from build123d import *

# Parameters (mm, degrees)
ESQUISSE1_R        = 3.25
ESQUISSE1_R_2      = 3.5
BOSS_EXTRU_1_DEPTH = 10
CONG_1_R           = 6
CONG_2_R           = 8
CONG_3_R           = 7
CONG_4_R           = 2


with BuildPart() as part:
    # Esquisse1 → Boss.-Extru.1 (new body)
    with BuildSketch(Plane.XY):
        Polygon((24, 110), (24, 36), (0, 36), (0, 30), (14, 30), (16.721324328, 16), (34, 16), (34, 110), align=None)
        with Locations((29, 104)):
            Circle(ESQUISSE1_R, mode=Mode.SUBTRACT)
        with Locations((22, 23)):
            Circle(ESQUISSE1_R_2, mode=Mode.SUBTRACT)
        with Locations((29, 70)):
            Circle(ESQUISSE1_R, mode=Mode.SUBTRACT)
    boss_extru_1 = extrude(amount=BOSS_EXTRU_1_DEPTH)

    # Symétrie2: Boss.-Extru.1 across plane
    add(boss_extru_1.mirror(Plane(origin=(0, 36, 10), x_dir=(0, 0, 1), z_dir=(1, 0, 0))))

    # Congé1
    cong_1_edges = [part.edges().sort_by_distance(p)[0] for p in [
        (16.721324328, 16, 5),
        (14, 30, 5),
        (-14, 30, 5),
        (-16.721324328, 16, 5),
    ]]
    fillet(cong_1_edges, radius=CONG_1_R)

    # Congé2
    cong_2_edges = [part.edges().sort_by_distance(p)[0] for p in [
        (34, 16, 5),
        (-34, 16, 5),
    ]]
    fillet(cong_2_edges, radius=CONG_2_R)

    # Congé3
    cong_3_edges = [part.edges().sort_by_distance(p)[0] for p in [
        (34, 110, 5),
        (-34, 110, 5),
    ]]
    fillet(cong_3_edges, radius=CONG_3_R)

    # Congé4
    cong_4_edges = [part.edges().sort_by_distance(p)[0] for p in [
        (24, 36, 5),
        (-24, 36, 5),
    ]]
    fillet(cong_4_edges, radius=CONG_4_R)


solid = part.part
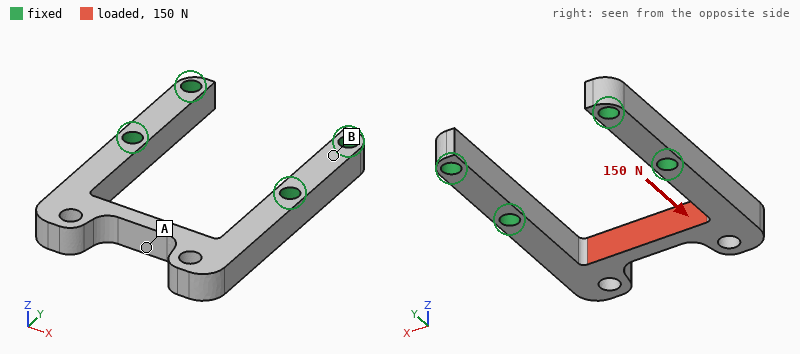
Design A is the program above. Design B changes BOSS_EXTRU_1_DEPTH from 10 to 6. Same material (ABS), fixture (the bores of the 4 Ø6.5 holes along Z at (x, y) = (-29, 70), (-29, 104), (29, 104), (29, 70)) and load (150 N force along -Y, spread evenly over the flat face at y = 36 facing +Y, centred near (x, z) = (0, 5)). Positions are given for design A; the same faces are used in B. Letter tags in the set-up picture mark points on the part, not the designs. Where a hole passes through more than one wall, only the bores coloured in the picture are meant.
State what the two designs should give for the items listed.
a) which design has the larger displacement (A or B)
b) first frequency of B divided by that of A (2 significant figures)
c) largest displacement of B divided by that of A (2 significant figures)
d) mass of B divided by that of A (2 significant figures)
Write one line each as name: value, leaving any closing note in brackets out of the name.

which design has the larger displacement: B
first frequency of B divided by that of A: 0.62
largest displacement of B divided by that of A: 1.7
mass of B divided by that of A: 0.60
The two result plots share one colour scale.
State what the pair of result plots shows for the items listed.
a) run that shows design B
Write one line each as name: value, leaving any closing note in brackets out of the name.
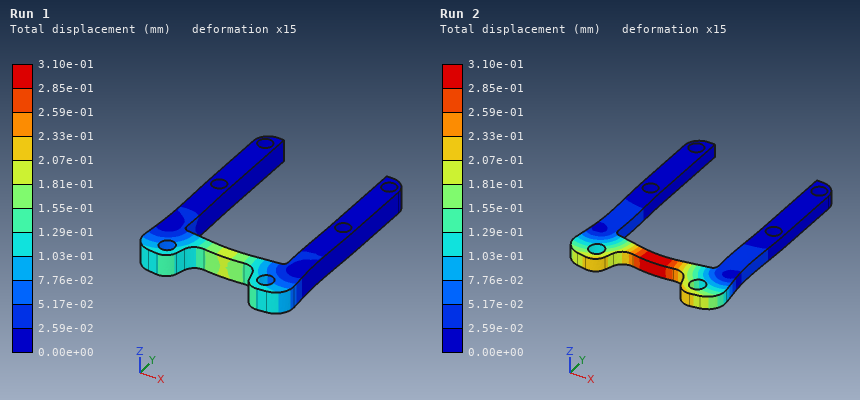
run that shows design B: Run 2
